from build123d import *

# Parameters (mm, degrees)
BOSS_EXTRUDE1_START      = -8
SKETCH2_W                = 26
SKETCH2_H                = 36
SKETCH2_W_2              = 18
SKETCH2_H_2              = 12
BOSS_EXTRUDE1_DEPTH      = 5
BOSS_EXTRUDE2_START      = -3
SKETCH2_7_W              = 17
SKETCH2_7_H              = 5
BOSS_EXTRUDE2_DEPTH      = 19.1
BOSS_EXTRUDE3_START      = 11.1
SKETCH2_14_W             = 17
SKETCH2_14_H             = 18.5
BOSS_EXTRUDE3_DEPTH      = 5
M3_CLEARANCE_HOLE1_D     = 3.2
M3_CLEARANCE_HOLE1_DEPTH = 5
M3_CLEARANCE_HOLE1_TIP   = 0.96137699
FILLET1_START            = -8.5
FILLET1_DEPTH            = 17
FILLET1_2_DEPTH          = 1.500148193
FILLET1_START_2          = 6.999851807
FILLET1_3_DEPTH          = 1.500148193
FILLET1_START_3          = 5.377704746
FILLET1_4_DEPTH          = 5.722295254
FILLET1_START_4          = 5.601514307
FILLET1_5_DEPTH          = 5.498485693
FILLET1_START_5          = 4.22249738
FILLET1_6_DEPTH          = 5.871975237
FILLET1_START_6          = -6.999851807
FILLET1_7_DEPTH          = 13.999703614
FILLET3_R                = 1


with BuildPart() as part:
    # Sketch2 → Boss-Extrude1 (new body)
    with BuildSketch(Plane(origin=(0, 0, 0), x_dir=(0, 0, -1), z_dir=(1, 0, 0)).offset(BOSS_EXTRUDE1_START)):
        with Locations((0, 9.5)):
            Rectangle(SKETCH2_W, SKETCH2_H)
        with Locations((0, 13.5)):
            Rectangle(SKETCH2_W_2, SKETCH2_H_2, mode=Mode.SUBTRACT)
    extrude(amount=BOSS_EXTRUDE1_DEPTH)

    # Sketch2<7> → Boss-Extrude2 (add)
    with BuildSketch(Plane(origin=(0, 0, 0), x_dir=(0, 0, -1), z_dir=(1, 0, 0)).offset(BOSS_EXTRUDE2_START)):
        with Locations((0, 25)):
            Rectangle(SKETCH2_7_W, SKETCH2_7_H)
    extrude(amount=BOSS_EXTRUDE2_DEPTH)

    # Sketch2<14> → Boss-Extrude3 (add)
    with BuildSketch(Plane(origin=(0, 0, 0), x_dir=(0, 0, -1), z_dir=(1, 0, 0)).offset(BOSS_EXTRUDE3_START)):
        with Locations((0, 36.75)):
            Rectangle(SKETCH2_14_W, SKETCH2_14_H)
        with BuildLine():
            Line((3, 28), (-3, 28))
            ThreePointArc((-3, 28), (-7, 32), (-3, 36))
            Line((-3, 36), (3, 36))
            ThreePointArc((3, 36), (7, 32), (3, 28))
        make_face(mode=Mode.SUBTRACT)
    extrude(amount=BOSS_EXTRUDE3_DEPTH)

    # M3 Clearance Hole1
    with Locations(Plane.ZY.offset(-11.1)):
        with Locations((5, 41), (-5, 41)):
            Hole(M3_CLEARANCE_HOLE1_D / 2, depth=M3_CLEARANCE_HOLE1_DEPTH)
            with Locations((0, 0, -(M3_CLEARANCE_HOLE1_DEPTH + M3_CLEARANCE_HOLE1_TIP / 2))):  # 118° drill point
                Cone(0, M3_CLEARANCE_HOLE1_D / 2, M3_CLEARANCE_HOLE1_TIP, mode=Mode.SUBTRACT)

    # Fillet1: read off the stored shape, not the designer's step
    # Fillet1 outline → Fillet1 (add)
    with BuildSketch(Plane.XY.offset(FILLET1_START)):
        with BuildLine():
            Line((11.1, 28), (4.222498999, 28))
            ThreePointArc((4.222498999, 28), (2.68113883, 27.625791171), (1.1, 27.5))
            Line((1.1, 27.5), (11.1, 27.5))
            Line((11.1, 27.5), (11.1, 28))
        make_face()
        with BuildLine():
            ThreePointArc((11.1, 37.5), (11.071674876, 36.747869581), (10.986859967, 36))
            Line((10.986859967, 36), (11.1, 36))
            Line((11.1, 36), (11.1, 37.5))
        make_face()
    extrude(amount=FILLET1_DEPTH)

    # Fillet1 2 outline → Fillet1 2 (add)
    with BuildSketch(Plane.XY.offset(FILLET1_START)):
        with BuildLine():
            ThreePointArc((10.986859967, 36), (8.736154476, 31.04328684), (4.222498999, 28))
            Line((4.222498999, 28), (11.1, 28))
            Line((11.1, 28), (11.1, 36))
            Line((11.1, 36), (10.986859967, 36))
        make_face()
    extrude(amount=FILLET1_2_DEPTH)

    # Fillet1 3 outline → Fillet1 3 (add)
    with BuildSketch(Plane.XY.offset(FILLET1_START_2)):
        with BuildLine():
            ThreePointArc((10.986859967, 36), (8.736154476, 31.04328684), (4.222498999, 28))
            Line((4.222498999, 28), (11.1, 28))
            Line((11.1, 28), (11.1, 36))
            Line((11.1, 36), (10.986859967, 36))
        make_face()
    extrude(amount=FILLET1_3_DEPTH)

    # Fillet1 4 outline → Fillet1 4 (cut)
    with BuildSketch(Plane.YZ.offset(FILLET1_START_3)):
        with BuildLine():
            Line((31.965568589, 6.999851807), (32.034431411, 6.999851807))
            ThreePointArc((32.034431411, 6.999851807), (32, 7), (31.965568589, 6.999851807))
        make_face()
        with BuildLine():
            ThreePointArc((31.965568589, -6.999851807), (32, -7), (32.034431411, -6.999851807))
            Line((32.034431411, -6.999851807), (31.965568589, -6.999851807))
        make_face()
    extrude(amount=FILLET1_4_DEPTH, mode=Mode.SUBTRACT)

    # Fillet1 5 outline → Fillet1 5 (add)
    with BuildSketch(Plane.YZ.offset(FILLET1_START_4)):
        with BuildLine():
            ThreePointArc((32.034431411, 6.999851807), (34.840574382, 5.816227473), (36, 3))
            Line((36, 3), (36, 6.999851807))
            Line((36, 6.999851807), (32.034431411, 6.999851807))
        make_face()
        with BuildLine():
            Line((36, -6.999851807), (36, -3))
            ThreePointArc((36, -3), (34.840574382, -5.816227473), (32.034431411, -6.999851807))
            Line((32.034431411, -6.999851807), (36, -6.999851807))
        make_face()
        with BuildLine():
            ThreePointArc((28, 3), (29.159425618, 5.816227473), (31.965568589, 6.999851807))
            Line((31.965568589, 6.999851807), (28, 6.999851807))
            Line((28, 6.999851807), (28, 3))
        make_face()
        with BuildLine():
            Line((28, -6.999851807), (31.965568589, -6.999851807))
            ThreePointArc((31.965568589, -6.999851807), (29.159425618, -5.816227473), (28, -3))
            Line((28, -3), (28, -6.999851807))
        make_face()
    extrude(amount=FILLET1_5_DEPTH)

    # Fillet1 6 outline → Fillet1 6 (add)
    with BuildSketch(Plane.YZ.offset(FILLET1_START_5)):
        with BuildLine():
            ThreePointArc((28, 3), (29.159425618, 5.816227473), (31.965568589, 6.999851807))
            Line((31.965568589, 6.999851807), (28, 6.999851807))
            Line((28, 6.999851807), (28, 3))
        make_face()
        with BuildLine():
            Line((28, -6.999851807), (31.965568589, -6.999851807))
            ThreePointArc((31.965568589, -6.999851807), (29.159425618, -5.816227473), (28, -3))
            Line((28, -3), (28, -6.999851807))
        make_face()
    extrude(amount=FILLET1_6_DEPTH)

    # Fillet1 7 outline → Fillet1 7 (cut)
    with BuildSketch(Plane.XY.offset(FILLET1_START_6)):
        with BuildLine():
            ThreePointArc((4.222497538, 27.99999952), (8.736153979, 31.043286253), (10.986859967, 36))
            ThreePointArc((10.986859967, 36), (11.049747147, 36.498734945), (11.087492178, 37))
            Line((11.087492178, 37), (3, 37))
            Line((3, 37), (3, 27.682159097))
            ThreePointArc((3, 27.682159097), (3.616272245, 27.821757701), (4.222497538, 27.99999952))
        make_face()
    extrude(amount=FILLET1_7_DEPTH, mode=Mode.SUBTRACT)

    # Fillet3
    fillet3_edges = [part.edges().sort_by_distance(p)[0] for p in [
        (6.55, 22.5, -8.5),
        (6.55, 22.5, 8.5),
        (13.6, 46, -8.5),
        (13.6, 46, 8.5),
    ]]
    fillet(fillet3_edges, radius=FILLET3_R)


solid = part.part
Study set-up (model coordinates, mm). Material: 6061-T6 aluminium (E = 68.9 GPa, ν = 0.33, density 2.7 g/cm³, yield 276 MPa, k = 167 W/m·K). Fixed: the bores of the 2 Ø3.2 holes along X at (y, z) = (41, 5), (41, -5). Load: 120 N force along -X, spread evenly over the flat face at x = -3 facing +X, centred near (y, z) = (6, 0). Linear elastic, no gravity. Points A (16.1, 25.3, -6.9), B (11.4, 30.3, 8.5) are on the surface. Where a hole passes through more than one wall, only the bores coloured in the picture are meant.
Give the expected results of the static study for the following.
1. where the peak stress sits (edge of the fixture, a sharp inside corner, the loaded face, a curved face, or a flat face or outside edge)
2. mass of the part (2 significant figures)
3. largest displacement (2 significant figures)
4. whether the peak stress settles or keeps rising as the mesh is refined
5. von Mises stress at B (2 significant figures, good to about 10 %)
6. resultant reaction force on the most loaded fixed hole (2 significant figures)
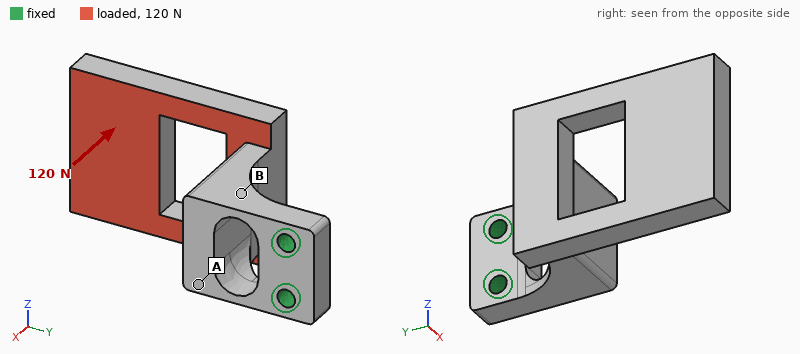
a sharp inside corner
17 g
0.59 mm
keeps rising
57 MPa
60 N
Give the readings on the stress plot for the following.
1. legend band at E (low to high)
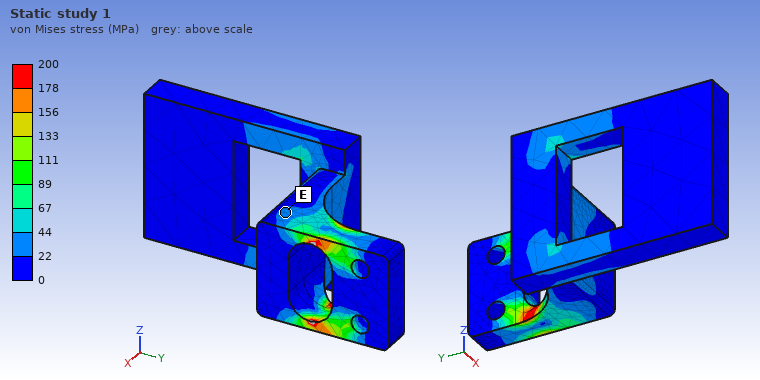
22 to 44 MPa
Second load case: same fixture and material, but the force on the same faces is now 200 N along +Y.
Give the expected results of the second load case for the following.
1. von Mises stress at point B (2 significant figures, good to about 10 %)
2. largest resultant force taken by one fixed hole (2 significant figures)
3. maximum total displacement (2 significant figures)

57 MPa
100 N
0.40 mm
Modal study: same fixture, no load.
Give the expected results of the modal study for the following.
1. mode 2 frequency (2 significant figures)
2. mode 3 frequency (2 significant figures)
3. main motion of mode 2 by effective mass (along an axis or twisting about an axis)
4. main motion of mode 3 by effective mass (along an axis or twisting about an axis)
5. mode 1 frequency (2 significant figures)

1900 Hz
3200 Hz
along Z
along Y
810 Hz
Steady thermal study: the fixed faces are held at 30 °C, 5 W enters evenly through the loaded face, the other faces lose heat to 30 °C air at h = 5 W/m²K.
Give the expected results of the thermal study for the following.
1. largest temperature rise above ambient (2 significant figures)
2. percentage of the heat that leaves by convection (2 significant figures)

28 K
5.4 %
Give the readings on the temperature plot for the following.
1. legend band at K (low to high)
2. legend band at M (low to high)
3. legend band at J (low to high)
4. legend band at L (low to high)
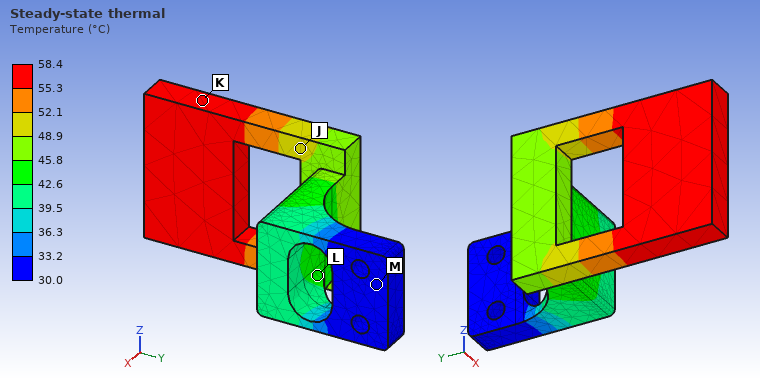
55.3 to 58.4 °C
30.0 to 33.2 °C
48.9 to 52.1 °C
42.6 to 45.8 °C
